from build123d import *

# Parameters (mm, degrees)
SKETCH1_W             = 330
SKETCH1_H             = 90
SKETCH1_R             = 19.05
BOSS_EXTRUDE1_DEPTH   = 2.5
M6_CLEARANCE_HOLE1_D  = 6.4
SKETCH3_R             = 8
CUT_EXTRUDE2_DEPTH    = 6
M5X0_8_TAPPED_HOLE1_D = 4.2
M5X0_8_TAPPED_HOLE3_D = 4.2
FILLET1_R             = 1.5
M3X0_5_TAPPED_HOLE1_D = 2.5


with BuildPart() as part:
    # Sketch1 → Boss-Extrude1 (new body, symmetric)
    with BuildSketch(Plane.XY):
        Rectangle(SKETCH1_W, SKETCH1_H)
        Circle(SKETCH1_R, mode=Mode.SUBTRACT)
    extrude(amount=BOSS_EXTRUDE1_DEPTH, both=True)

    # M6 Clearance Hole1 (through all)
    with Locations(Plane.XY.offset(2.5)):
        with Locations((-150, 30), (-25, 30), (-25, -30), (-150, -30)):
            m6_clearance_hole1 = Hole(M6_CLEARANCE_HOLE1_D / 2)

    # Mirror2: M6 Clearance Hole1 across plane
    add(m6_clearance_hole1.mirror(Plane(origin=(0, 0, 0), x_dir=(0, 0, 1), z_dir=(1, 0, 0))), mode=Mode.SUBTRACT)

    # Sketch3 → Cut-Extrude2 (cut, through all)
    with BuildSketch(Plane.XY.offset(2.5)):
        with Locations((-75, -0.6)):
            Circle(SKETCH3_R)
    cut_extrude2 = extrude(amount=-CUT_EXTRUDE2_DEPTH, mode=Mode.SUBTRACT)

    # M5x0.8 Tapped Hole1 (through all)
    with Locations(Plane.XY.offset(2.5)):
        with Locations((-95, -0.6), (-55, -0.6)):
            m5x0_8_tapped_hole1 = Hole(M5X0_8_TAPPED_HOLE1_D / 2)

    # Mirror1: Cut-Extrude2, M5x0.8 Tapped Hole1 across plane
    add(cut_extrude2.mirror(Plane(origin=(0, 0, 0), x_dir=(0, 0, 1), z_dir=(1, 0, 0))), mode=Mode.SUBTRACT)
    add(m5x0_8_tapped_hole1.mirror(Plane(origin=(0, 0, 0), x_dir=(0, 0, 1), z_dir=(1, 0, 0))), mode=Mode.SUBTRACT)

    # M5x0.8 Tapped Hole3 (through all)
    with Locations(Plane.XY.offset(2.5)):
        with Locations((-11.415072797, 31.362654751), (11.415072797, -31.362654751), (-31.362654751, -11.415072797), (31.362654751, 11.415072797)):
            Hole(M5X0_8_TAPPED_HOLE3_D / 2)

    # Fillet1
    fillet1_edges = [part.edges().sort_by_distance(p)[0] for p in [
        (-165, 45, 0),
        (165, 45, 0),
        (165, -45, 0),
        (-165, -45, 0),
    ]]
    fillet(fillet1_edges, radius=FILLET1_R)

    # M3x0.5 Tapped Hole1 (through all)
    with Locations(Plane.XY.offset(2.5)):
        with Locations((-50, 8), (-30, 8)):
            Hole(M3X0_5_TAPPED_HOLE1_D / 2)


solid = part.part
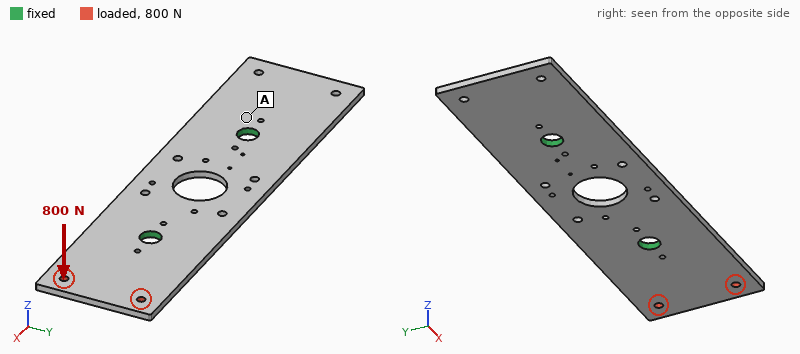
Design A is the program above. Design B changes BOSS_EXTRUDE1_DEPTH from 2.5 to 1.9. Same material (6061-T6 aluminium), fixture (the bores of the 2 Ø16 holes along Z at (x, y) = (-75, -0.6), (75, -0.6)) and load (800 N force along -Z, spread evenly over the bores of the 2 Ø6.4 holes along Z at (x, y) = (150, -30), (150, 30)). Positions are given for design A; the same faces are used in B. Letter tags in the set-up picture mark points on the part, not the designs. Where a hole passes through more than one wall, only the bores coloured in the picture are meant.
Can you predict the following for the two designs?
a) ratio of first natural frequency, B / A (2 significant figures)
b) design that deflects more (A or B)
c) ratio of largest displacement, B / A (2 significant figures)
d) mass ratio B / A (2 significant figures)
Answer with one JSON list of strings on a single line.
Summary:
["0.77", "B", "2.3", "0.76"]
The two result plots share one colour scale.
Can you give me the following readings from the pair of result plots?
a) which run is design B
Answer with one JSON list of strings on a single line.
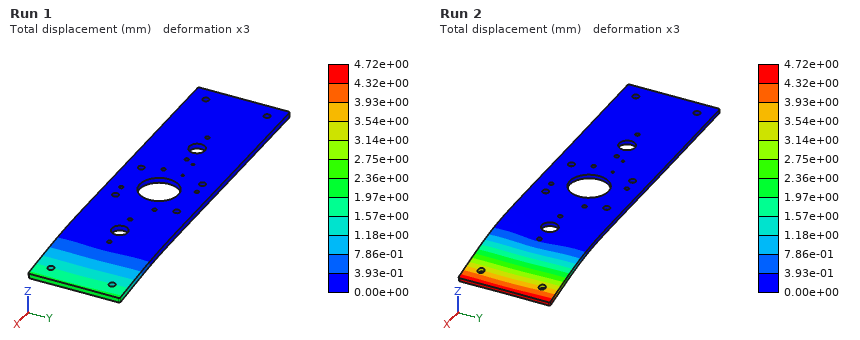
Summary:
["Run 2"]
